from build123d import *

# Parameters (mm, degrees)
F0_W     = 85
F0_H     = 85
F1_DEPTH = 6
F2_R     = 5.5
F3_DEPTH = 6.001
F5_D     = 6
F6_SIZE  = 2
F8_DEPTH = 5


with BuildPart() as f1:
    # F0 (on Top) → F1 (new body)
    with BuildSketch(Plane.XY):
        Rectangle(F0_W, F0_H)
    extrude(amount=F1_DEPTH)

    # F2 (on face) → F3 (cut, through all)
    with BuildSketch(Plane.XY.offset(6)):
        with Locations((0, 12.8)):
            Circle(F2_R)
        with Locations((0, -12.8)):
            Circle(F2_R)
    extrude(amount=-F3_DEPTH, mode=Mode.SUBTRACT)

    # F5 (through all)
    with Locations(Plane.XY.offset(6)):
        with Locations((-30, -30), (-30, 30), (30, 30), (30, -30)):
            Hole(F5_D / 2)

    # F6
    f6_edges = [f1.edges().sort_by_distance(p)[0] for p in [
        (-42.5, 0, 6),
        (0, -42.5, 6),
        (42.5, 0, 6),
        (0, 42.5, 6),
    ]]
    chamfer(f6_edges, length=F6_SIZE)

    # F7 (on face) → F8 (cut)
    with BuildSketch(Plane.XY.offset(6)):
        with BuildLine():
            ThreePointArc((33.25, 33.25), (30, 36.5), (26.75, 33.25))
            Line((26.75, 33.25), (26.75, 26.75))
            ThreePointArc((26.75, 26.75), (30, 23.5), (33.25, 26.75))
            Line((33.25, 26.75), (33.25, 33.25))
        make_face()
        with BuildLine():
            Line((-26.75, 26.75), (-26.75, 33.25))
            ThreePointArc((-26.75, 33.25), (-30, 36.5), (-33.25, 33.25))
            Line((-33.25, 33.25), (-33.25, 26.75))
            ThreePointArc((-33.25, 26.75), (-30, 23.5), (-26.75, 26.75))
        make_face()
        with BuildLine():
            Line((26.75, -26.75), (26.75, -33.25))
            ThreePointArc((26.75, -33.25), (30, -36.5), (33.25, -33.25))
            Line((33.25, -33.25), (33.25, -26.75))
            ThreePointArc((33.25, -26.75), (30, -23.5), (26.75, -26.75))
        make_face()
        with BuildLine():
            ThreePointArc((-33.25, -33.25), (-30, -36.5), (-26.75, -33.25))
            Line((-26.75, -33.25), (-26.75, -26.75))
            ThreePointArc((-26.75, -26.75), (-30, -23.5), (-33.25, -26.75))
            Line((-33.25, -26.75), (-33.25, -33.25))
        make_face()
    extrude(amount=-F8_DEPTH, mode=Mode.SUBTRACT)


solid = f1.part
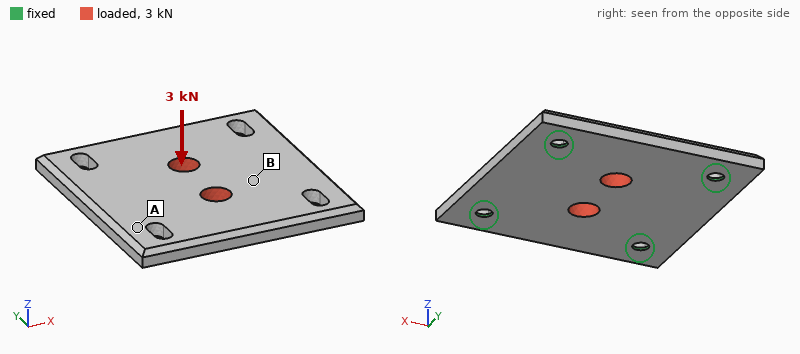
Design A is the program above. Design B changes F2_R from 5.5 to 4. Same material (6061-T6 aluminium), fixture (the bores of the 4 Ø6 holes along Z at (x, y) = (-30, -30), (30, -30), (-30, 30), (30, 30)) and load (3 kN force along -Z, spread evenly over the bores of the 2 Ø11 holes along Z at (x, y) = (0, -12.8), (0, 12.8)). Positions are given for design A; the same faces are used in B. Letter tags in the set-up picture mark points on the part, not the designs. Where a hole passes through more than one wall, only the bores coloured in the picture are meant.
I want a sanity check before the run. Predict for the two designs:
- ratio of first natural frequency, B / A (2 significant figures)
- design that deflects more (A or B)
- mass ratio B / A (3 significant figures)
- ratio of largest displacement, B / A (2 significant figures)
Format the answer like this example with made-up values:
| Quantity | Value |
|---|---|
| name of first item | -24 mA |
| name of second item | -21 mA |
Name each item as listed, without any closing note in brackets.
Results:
| Quantity | Value |
|---|---|
| ratio of first natural frequency, B / A | 1.0 |
| design that deflects more | A |
| mass ratio B / A | 1.01 |
| ratio of largest displacement, B / A | 0.92 |
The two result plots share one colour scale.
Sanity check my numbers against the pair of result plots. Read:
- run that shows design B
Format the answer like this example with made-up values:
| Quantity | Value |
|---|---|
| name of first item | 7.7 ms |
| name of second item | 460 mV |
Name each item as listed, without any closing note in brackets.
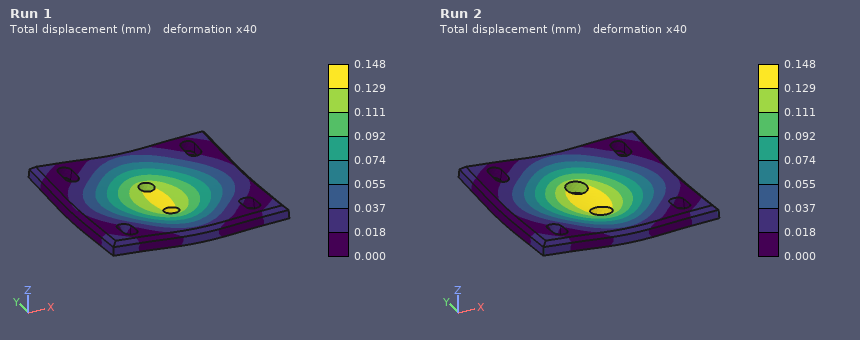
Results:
| Quantity | Value |
|---|---|
| run that shows design B | Run 1 |
